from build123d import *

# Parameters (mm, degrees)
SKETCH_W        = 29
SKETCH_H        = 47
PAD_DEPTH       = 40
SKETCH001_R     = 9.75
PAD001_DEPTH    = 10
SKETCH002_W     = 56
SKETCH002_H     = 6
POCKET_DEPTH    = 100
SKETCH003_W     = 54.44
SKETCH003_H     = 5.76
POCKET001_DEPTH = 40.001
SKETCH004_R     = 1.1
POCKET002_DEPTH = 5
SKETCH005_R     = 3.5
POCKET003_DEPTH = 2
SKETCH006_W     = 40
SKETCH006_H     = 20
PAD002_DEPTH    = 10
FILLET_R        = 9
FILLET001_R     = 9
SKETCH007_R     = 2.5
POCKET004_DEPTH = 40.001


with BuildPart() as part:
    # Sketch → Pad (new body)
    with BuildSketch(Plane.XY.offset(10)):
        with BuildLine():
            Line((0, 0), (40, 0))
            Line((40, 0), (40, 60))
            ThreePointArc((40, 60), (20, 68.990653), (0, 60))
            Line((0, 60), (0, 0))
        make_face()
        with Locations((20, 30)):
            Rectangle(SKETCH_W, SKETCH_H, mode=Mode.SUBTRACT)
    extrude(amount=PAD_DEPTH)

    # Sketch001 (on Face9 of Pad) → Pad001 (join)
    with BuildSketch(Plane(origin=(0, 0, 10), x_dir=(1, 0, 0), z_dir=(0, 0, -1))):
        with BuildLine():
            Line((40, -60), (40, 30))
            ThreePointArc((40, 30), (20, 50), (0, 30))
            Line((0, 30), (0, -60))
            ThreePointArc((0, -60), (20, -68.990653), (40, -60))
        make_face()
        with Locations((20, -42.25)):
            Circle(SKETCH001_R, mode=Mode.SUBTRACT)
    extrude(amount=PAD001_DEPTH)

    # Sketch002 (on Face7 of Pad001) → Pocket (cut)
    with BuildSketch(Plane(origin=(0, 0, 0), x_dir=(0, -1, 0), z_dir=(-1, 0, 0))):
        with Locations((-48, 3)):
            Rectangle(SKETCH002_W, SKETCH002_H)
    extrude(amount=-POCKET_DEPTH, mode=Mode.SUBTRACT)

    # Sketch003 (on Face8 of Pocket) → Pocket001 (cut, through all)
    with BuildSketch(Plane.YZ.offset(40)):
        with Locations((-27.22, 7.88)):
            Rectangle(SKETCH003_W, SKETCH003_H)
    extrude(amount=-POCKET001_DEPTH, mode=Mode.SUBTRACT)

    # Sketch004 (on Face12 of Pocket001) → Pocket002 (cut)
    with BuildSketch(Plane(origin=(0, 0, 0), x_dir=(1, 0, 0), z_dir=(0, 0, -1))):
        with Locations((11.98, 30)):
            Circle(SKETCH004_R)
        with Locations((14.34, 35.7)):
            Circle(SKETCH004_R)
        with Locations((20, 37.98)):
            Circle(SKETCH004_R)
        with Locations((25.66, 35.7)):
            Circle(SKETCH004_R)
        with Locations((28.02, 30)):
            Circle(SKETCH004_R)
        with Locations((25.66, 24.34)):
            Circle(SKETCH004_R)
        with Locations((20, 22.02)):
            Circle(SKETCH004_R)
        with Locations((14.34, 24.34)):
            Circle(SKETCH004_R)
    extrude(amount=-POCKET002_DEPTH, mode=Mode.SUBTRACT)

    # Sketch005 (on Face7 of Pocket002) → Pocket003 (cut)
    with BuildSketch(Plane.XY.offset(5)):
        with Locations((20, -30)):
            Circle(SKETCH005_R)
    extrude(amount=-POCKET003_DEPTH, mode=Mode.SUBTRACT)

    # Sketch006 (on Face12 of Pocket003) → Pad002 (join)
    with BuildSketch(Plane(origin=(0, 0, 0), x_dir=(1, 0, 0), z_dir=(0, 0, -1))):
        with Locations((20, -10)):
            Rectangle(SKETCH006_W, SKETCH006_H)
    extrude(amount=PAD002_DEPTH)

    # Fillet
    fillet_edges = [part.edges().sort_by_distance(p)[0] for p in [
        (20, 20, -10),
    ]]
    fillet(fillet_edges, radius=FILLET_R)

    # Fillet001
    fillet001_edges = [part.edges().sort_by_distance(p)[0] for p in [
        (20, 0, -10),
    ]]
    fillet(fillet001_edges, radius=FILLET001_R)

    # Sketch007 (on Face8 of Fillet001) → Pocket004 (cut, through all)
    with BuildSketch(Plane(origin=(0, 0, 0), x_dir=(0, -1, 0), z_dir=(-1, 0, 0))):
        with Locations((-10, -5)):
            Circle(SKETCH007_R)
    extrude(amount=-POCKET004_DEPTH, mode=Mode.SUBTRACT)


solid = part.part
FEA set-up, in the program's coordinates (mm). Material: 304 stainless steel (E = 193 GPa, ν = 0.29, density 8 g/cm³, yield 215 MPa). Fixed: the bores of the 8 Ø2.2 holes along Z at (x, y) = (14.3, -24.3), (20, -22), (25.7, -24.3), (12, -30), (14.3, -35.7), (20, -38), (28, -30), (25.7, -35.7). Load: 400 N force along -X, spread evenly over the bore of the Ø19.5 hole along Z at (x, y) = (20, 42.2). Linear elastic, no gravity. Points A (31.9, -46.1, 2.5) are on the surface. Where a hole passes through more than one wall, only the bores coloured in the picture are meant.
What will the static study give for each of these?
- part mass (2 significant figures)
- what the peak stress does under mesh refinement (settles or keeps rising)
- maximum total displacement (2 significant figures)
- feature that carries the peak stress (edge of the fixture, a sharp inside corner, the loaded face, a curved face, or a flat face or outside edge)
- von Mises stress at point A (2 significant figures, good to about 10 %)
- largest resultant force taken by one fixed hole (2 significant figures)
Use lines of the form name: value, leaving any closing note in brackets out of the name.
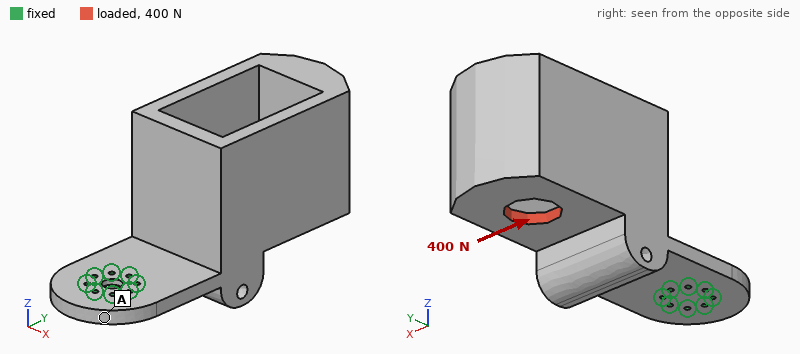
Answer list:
part mass: 640 g
what the peak stress does under mesh refinement: keeps rising
maximum total displacement: 32 µm
feature that carries the peak stress: edge of the fixture
von Mises stress at point A: 2.5 MPa
largest resultant force taken by one fixed hole: 570 N
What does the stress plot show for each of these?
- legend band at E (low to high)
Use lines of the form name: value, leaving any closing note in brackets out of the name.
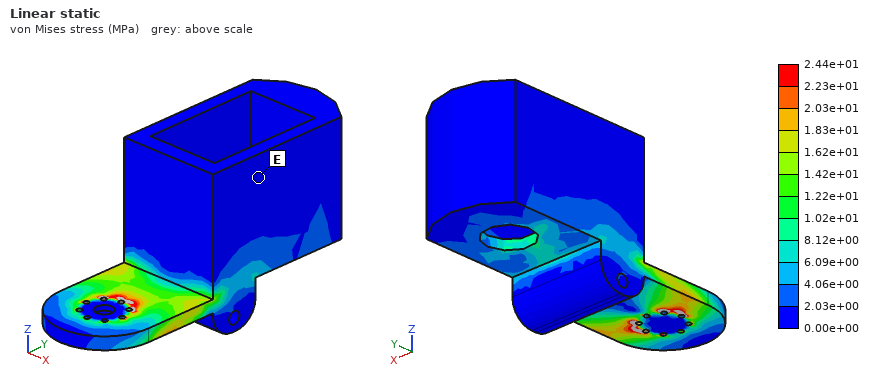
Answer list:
legend band at E: 0.00e+00 to 2.03e+00 MPa
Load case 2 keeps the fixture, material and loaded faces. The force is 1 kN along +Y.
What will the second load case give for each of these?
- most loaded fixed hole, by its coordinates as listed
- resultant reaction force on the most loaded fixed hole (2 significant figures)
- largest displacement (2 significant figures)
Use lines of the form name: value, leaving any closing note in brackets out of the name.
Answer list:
most loaded fixed hole, by its coordinates as listed: (20, -22)
resultant reaction force on the most loaded fixed hole: 310 N
largest displacement: 0.16 mm
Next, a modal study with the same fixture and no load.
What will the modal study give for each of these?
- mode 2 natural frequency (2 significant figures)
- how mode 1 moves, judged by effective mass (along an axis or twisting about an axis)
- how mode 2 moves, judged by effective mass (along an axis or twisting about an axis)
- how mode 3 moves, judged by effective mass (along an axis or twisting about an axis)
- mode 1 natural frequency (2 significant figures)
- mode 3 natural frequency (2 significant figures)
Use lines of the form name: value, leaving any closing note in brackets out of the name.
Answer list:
mode 2 natural frequency: 600 Hz
how mode 1 moves, judged by effective mass: along Z
how mode 2 moves, judged by effective mass: along X
how mode 3 moves, judged by effective mass: along X
mode 1 natural frequency: 210 Hz
mode 3 natural frequency: 1700 Hz
